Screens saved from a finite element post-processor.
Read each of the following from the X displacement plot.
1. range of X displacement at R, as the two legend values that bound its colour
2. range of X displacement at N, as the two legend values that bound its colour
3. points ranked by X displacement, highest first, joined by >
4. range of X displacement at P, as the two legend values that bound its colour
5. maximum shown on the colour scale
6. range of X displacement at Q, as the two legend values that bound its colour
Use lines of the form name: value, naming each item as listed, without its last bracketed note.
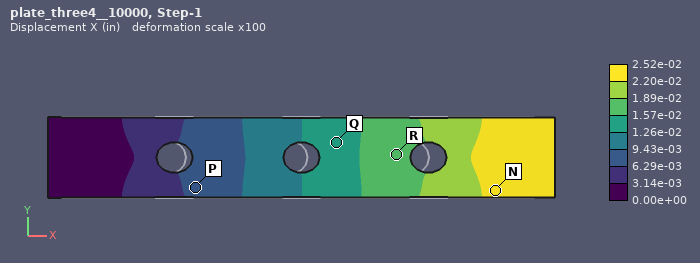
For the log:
range of X displacement at R, as the two legend values that bound its colour: 1.57e-02 to 1.89e-02 in
range of X displacement at N, as the two legend values that bound its colour: 2.20e-02 to 2.52e-02 in
points ranked by X displacement, highest first, joined by >: N > R > Q > P
range of X displacement at P, as the two legend values that bound its colour: 6.29e-03 to 9.43e-03 in
maximum shown on the colour scale: 2.52e-02 in
range of X displacement at Q, as the two legend values that bound its colour: 1.26e-02 to 1.57e-02 in
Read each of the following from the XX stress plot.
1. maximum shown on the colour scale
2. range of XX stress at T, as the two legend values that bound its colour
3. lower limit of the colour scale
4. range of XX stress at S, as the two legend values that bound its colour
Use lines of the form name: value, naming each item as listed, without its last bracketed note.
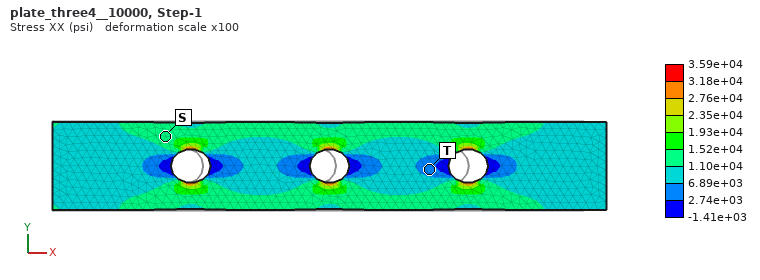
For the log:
maximum shown on the colour scale: 3.59e+04 psi
range of XX stress at T, as the two legend values that bound its colour: 2.74e+03 to 6.89e+03 psi
lower limit of the colour scale: -1.41e+03 psi
range of XX stress at S, as the two legend values that bound its colour: 1.10e+04 to 1.52e+04 psi
